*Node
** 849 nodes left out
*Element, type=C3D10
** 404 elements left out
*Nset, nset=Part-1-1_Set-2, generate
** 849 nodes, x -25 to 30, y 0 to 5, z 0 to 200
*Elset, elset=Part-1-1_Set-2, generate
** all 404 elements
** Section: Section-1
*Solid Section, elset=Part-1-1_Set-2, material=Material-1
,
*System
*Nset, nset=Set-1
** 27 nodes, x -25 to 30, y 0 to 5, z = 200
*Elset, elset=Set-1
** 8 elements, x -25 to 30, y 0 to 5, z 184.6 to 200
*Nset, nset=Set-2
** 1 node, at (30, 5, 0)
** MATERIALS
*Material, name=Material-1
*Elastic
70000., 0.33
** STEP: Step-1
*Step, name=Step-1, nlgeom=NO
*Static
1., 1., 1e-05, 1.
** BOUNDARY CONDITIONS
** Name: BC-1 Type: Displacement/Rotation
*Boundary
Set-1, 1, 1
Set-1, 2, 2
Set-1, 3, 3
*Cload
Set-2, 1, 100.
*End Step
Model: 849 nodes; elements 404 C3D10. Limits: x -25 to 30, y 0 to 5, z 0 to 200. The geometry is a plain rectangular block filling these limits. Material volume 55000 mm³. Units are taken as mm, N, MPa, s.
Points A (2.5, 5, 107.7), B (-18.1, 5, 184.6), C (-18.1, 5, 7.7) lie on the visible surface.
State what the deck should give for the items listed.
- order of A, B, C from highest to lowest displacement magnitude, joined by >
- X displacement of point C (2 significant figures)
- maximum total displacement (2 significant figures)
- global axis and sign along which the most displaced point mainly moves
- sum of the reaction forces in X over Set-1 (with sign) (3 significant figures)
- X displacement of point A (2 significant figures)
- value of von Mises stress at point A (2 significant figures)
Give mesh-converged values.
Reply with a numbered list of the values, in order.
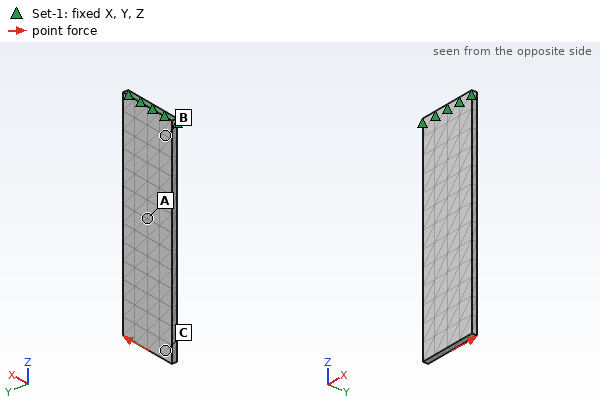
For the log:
1. C > A > B
2. 0.056 mm
3. 0.069 mm
4. +X
5. -100 N
6. 0.017 mm
7. 1.9 MPa
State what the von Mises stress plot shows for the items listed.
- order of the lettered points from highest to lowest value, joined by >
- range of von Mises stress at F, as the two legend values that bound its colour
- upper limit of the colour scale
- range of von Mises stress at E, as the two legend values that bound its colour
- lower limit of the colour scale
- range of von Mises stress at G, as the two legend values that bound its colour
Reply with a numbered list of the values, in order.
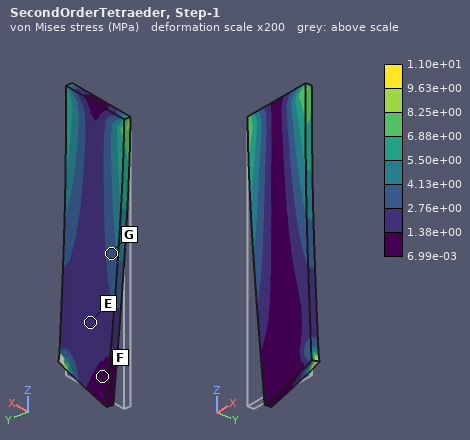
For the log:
1. G > E > F
2. 6.99e-03 to 1.38e+00 MPa
3. 1.10e+01 MPa
4. 1.38e+00 to 2.76e+00 MPa
5. 6.99e-03 MPa
6. 2.76e+00 to 4.13e+00 MPa
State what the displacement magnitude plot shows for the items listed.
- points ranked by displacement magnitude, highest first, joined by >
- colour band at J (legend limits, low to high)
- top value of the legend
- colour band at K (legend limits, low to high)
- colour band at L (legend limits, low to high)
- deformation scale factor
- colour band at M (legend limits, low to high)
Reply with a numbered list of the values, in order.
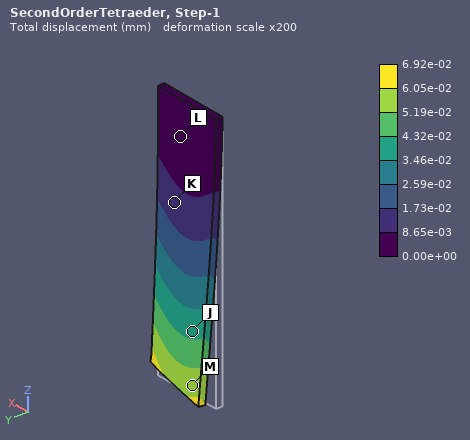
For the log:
1. M > J > K > L
2. 3.46e-02 to 4.32e-02 mm
3. 6.92e-02 mm
4. 8.65e-03 to 1.73e-02 mm
5. 0.00e+00 to 8.65e-03 mm
6. 200
7. 5.19e-02 to 6.05e-02 mm
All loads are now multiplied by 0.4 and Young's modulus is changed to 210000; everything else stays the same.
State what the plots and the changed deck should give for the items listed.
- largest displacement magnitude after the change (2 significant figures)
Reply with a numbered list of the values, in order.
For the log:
1. 0.0092 mm
